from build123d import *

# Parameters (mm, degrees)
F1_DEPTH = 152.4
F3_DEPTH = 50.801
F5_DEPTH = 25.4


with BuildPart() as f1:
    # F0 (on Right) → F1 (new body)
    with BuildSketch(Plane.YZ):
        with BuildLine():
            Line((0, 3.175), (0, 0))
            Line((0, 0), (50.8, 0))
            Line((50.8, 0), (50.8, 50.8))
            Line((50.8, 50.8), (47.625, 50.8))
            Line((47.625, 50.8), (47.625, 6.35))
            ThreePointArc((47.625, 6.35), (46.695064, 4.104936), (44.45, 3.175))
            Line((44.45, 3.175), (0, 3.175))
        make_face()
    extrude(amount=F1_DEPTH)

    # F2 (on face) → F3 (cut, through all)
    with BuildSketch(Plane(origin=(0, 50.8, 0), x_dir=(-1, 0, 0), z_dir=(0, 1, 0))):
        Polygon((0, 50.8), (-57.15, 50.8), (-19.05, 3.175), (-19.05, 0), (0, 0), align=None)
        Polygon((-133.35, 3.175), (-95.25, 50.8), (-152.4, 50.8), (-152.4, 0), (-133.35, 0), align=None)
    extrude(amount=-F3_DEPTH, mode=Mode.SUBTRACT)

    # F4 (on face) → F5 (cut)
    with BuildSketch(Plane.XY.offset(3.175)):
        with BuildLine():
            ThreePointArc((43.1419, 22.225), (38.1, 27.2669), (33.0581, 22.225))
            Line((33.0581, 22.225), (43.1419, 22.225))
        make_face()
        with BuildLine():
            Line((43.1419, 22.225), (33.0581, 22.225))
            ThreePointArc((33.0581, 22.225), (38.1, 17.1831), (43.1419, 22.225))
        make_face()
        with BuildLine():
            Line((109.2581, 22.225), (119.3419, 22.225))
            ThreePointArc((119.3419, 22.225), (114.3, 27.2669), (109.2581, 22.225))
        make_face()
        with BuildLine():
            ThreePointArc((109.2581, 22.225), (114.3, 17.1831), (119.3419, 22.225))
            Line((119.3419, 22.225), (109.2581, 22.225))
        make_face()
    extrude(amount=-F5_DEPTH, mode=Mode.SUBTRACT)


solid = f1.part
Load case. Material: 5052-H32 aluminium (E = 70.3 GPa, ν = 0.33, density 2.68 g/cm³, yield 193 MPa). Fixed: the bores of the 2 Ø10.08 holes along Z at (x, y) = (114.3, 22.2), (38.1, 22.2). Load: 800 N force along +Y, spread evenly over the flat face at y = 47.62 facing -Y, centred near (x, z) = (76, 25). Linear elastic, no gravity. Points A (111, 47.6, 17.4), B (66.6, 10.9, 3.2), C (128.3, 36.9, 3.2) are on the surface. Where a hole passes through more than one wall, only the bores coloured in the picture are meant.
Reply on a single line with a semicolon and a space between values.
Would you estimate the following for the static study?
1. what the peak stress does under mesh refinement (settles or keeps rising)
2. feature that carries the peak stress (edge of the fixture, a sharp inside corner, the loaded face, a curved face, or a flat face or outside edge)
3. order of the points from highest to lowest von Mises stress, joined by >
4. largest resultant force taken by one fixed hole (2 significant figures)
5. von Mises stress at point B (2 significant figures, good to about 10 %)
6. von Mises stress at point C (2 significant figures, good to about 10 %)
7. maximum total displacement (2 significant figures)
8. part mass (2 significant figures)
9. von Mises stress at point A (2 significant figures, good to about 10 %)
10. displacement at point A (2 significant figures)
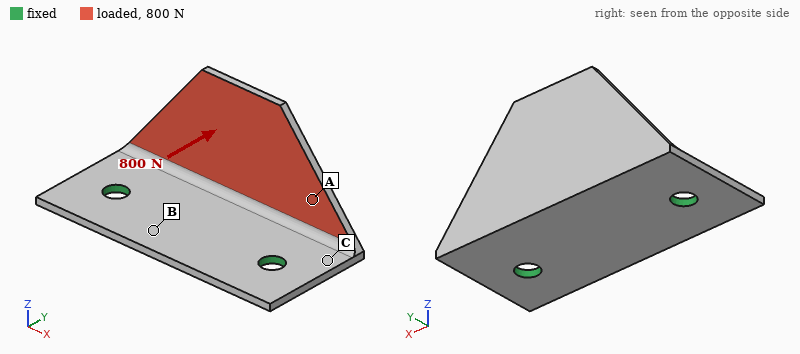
keeps rising; edge of the fixture; C > A > B; 410 N; 19 MPa; 86 MPa; 1.6 mm; 80 g; 50 MPa; 0.44 mm
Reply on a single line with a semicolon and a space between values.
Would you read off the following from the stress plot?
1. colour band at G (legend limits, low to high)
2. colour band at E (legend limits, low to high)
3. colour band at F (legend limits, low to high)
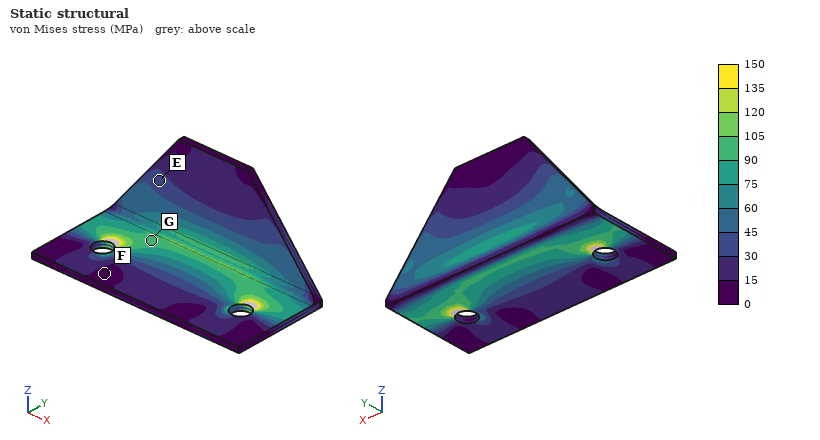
90 to 105 MPa; 30 to 45 MPa; 0 to 15 MPa
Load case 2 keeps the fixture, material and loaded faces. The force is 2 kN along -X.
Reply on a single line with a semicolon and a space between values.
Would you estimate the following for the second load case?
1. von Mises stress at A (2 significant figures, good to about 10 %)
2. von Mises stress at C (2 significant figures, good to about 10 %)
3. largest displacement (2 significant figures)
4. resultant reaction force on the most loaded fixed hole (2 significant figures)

47 MPa; 56 MPa; 0.38 mm; 1.3 kN
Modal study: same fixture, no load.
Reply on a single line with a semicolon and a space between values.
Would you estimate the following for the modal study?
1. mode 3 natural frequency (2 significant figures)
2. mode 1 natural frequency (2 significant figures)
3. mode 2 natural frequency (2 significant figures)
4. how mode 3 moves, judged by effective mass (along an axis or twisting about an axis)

2100 Hz; 820 Hz; 1900 Hz; along Z
